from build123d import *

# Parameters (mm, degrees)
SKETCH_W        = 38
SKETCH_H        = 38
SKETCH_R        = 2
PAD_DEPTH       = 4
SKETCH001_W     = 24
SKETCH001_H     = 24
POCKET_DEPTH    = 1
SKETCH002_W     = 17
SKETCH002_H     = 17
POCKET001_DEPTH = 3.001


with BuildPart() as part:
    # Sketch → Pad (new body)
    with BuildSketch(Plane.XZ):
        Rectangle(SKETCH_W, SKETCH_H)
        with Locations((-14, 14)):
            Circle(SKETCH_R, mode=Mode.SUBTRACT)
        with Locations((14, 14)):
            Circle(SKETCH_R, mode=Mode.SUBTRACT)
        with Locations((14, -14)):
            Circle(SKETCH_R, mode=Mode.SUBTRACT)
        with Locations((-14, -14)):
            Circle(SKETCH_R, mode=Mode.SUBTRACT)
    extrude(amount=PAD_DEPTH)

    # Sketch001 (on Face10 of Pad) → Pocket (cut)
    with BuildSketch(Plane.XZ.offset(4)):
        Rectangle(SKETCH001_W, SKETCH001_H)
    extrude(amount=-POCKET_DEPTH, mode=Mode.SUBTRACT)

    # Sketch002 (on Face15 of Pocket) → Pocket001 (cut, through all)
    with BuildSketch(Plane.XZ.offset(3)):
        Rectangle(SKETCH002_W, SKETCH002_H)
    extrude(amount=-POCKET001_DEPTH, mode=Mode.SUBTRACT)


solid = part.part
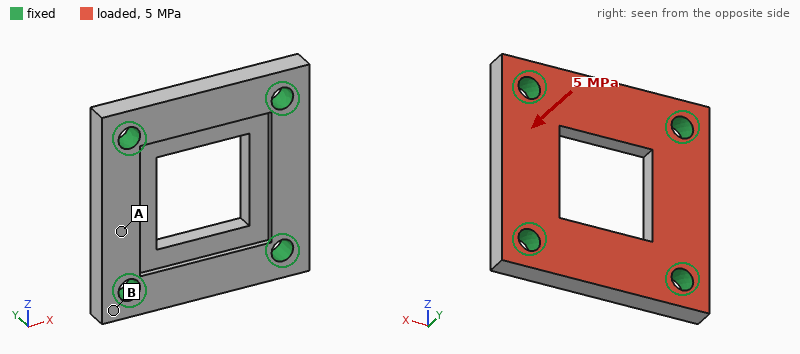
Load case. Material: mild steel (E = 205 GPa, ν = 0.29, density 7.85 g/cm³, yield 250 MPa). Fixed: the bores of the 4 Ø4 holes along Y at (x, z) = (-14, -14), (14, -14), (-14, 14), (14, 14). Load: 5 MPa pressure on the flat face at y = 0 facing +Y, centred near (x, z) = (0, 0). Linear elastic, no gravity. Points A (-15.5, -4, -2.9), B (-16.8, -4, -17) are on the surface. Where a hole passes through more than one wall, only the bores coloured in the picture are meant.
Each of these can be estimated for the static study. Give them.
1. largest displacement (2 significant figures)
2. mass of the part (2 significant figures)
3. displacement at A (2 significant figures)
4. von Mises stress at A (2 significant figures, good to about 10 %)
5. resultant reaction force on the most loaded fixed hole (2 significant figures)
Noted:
11 µm
32 g
6.7 µm
49 MPa
1.4 kN
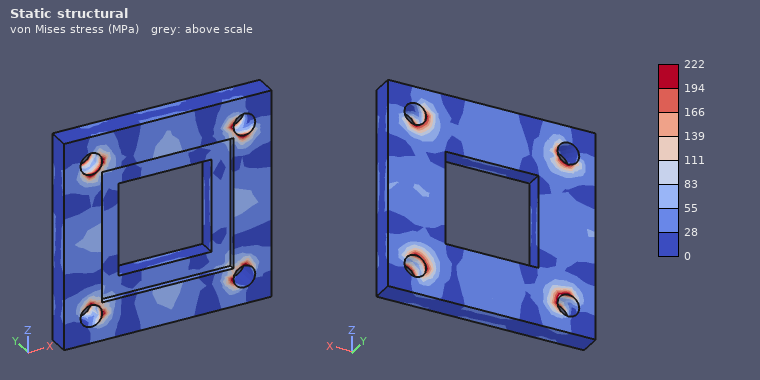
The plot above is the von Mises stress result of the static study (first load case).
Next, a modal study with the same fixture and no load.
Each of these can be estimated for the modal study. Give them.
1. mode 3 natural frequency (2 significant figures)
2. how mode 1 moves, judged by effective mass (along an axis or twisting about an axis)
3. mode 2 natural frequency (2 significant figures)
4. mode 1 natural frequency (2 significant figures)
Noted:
27 kHz
along Y
27 kHz
26 kHz
